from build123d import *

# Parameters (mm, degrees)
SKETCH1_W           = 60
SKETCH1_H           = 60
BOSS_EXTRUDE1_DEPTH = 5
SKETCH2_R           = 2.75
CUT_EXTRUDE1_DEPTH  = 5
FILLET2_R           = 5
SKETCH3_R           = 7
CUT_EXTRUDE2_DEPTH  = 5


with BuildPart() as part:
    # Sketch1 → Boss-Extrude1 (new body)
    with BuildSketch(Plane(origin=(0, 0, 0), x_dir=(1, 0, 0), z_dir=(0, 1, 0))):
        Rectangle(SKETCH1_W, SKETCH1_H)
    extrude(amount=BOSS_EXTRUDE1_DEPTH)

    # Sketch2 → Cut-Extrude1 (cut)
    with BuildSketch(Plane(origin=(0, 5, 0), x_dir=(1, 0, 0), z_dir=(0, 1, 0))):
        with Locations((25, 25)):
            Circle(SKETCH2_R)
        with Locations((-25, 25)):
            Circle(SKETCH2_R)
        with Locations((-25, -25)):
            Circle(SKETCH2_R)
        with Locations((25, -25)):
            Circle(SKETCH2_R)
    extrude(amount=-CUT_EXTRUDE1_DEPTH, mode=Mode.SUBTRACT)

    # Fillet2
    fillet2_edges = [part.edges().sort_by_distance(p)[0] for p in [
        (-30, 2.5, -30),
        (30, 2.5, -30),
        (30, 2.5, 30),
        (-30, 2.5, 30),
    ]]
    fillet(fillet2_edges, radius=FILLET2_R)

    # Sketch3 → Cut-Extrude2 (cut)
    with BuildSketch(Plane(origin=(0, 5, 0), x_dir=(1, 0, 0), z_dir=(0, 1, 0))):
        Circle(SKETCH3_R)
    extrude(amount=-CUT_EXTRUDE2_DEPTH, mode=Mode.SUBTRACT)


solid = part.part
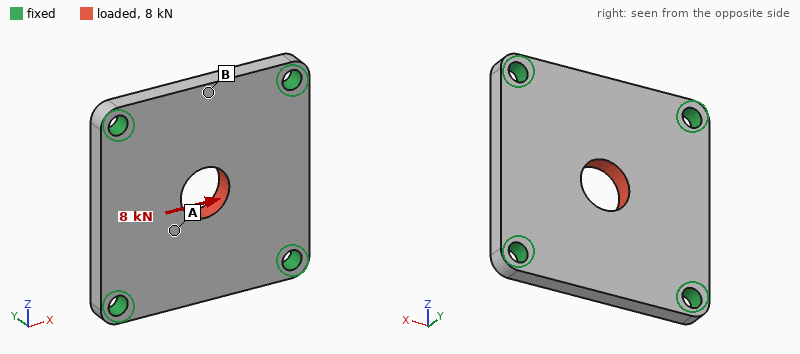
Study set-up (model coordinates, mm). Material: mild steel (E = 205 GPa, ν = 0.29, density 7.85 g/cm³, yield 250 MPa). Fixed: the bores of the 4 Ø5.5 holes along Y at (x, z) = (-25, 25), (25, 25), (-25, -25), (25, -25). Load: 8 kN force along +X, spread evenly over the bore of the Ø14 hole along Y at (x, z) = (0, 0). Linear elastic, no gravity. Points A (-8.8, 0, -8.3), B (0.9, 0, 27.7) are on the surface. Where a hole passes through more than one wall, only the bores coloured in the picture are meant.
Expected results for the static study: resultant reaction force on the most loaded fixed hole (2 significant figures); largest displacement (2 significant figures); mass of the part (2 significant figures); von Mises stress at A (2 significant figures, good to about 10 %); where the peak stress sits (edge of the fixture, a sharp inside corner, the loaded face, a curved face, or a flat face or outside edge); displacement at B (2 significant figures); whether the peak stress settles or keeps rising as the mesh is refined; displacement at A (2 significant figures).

2.3 kN
5.7 µm
130 g
30 MPa
edge of the fixture
1.4 µm
keeps rising
4.1 µm
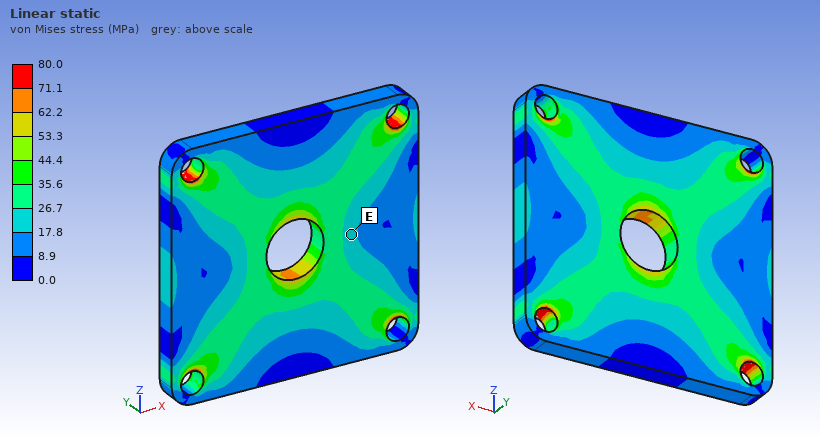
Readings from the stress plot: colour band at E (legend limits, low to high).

17.8 to 26.7 MPa
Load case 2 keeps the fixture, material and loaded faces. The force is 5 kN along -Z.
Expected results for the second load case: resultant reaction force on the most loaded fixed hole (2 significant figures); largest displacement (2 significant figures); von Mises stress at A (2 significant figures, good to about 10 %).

1.4 kN
3.5 µm
19 MPa
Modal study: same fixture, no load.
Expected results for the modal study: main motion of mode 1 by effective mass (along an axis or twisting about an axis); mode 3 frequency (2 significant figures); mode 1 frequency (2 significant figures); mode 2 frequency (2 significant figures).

along Y
12 kHz
7200 Hz
12 kHz
